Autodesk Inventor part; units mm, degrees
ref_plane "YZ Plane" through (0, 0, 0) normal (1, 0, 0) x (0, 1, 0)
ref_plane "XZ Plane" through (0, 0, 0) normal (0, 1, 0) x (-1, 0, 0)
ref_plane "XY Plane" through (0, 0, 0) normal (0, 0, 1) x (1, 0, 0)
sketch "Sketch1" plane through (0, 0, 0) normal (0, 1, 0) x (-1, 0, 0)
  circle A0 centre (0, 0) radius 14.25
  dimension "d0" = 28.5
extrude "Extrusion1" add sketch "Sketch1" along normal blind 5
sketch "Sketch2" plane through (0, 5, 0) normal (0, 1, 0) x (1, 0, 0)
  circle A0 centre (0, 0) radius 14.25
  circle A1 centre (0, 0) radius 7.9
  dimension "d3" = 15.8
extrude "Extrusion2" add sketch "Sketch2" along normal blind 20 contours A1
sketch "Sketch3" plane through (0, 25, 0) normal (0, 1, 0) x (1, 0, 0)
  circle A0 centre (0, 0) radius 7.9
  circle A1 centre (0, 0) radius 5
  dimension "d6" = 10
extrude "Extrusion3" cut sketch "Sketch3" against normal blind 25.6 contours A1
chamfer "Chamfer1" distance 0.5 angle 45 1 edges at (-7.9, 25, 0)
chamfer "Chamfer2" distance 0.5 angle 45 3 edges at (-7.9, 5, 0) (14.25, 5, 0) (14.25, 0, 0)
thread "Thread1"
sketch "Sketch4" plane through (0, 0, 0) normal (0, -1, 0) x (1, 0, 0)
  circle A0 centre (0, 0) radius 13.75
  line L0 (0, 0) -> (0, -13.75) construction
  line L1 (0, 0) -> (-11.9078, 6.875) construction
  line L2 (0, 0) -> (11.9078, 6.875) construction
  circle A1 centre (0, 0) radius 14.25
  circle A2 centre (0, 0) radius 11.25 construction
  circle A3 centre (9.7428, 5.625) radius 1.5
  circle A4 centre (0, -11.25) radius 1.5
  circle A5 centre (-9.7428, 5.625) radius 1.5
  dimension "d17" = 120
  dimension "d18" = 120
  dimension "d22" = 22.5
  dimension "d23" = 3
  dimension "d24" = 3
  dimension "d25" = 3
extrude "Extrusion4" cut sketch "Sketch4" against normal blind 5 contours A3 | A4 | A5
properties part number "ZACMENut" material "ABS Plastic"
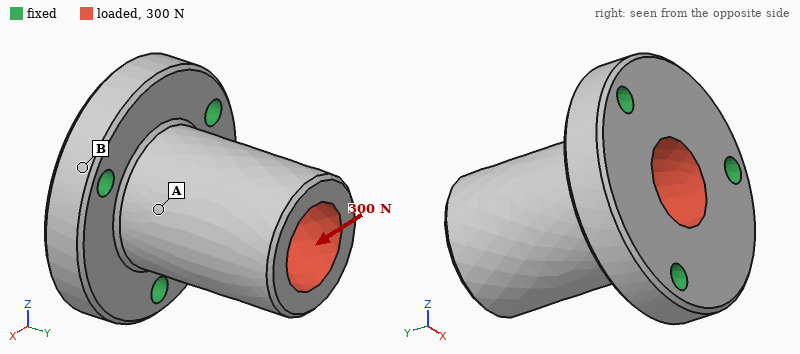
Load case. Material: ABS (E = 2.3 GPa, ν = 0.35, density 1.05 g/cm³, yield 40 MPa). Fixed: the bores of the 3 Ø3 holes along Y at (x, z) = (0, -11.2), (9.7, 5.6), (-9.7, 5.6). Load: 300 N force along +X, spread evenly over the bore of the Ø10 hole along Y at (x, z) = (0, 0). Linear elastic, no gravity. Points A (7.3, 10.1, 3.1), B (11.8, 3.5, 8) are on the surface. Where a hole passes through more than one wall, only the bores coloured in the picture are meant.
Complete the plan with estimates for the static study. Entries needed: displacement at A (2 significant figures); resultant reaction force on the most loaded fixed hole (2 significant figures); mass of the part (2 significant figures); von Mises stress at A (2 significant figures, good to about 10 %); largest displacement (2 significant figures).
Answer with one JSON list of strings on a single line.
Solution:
["0.061 mm", "180 N", "5.3 g", "3.9 MPa", "0.17 mm"]
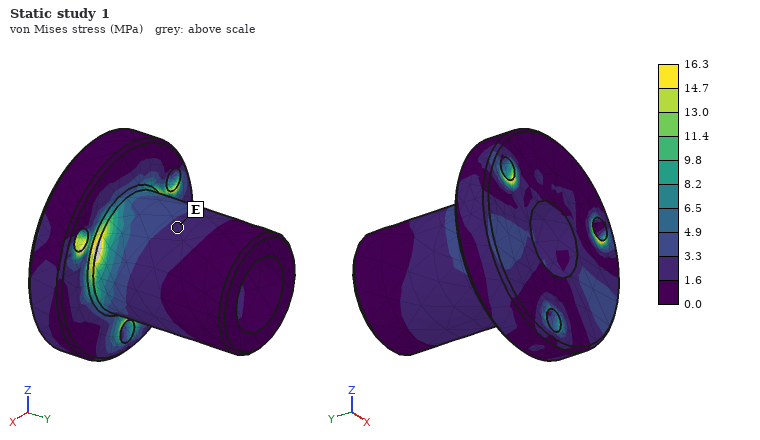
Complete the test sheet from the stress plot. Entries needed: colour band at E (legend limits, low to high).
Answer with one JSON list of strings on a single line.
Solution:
["1.6 to 3.3 MPa"]
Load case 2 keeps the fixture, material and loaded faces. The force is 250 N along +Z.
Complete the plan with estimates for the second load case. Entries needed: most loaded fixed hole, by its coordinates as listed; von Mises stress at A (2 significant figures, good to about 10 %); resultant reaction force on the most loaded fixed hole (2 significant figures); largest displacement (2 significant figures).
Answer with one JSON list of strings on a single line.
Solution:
["(0, -11.2)", "2.9 MPa", "170 N", "0.14 mm"]
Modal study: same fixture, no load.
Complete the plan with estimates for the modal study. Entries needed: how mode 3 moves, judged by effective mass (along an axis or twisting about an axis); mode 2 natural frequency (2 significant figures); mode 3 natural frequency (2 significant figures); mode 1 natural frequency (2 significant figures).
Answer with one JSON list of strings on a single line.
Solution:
["along Y", "4500 Hz", "9700 Hz", "4500 Hz"]
